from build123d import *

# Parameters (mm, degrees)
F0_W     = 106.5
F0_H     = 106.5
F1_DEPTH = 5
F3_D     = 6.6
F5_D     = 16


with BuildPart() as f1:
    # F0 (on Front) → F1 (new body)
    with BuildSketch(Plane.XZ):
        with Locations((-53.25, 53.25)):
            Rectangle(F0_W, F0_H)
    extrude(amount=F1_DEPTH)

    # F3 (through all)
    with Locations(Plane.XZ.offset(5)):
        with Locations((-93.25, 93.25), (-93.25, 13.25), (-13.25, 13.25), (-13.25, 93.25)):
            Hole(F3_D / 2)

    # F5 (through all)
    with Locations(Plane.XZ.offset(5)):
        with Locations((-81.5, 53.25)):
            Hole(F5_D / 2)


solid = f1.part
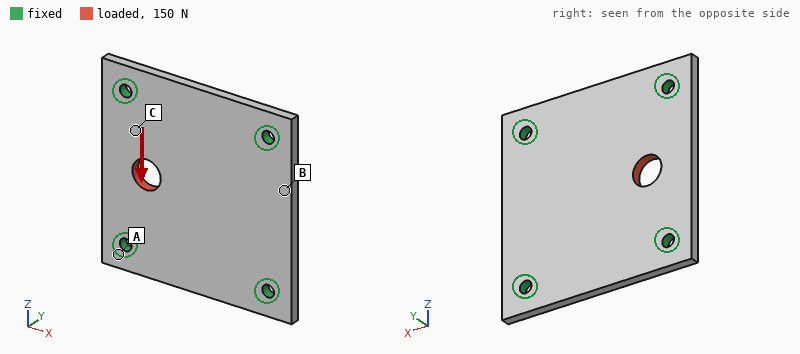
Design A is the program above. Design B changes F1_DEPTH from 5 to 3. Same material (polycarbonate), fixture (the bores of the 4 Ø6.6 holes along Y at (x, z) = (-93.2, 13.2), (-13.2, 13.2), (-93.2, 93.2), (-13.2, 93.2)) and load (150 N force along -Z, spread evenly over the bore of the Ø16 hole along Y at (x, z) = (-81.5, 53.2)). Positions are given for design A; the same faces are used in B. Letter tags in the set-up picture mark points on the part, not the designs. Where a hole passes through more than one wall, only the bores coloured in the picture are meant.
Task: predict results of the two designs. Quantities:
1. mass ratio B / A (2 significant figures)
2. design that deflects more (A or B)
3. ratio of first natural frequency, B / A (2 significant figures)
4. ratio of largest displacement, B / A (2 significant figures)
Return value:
0.60
B
0.63
1.7
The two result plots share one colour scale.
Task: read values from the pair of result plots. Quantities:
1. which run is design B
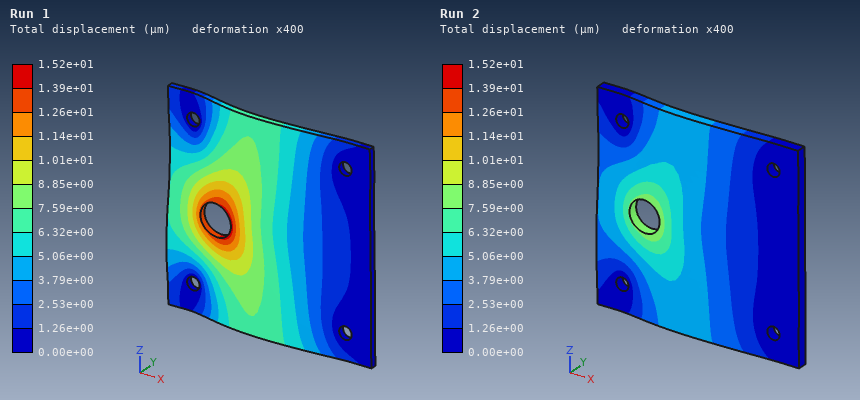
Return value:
Run 1
